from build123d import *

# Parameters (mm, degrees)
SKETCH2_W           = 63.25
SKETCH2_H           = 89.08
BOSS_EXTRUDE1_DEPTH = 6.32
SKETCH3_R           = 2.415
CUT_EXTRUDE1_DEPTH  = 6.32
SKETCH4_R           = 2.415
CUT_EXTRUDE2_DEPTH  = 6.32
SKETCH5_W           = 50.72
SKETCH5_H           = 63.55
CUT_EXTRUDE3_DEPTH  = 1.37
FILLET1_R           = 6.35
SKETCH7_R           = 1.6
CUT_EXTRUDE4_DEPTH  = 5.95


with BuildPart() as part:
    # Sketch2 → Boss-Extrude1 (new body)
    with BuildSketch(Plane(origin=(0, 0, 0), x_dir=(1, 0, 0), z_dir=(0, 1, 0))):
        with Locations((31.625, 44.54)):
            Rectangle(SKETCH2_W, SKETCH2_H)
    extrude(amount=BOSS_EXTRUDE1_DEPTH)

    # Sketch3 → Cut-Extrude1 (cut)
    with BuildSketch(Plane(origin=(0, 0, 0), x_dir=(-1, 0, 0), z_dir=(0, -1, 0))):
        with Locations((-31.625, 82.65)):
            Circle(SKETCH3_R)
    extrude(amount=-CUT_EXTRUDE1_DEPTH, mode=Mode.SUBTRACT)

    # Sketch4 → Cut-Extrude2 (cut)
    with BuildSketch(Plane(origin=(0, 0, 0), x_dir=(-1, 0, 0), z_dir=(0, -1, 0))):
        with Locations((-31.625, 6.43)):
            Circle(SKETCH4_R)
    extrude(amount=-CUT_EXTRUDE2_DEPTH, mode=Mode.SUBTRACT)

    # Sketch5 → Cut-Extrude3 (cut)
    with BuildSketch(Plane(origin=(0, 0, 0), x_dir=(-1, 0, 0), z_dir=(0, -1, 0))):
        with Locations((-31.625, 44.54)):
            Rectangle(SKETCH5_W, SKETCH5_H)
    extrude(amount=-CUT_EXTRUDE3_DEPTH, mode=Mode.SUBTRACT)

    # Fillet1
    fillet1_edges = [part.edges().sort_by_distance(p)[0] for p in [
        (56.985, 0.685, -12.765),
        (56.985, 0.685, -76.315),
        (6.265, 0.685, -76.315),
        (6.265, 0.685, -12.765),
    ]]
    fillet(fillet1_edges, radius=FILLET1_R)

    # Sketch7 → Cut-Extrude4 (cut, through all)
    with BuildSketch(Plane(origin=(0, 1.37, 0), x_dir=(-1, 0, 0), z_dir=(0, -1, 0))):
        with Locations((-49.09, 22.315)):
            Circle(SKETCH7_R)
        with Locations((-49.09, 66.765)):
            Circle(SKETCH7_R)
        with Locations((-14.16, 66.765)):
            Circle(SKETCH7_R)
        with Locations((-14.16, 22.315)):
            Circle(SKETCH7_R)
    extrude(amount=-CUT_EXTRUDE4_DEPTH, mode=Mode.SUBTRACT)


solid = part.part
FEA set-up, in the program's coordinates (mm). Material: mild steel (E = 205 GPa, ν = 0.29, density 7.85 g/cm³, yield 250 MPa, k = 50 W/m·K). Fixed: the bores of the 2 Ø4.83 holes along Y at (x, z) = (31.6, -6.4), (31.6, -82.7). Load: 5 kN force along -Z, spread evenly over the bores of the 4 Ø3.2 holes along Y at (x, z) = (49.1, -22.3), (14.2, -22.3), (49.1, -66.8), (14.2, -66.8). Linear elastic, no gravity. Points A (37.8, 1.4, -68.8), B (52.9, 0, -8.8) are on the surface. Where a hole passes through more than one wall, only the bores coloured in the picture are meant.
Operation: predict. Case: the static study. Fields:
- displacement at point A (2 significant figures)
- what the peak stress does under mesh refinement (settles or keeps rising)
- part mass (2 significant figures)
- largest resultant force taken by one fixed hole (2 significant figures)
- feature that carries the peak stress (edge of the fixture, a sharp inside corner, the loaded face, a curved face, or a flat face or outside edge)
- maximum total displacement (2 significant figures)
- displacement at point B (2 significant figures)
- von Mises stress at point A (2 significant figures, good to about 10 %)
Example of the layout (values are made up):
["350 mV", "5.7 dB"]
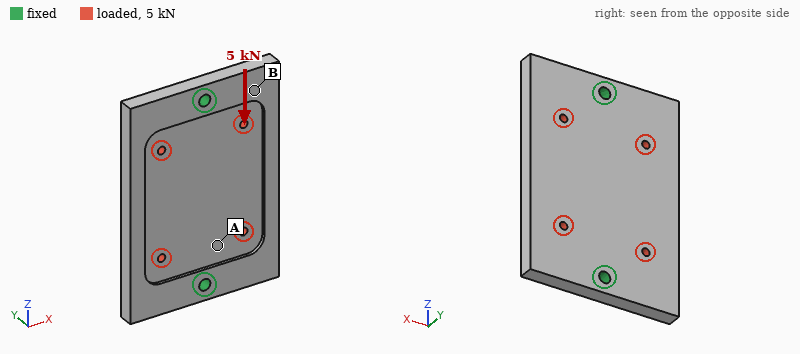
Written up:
["1.6 µm", "keeps rising", "240 g", "2.5 kN", "edge of the fixture", "3.2 µm", "2.4 µm", "17 MPa"]
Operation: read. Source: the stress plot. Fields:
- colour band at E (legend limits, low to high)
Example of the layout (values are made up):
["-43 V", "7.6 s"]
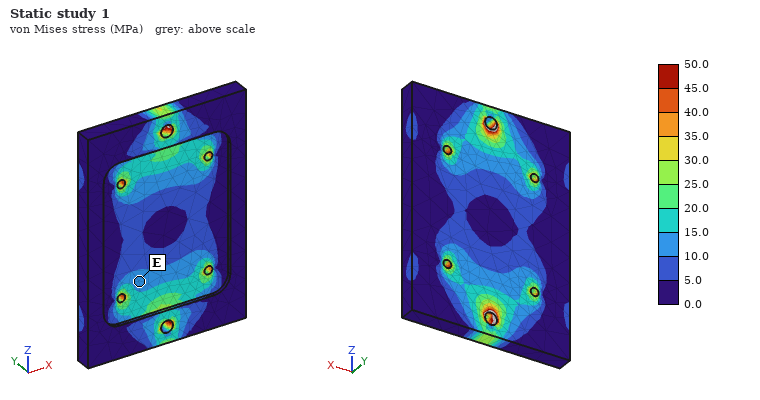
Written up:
["10.0 to 15.0 MPa"]
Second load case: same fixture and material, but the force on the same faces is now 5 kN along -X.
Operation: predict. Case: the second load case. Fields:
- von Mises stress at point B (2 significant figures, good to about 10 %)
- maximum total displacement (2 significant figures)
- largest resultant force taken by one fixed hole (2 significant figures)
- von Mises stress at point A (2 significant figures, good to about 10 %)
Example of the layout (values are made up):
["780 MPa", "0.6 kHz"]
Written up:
["6.1 MPa", "5.0 µm", "2.5 kN", "12 MPa"]
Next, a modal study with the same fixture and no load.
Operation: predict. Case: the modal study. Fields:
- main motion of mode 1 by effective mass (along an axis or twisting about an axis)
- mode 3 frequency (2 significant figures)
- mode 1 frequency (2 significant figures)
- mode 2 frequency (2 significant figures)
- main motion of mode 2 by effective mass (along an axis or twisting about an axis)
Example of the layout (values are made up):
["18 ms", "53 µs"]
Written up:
["twisting about Z", "5400 Hz", "2700 Hz", "3300 Hz", "along Y"]
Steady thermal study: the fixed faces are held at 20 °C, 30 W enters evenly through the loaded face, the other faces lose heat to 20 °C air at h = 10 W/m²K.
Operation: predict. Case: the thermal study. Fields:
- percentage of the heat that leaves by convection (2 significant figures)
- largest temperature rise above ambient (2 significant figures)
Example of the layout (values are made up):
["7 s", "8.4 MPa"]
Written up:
["9.4 %", "33 K"]
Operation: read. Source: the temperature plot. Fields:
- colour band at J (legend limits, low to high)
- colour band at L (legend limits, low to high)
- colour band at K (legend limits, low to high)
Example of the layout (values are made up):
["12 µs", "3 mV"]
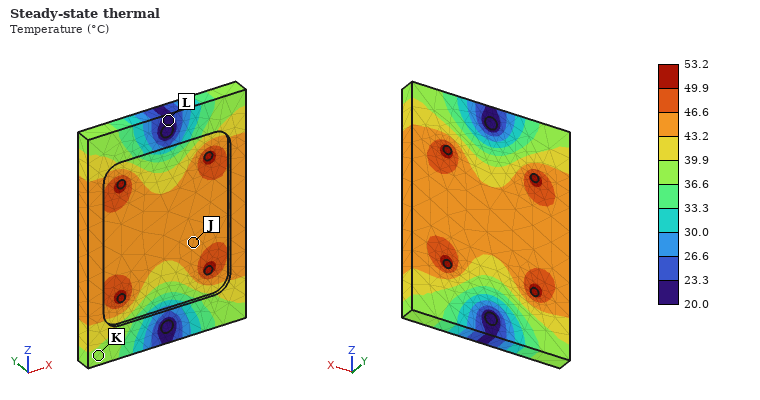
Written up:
["43.2 to 46.6 °C", "20.0 to 23.3 °C", "36.6 to 39.9 °C"]
